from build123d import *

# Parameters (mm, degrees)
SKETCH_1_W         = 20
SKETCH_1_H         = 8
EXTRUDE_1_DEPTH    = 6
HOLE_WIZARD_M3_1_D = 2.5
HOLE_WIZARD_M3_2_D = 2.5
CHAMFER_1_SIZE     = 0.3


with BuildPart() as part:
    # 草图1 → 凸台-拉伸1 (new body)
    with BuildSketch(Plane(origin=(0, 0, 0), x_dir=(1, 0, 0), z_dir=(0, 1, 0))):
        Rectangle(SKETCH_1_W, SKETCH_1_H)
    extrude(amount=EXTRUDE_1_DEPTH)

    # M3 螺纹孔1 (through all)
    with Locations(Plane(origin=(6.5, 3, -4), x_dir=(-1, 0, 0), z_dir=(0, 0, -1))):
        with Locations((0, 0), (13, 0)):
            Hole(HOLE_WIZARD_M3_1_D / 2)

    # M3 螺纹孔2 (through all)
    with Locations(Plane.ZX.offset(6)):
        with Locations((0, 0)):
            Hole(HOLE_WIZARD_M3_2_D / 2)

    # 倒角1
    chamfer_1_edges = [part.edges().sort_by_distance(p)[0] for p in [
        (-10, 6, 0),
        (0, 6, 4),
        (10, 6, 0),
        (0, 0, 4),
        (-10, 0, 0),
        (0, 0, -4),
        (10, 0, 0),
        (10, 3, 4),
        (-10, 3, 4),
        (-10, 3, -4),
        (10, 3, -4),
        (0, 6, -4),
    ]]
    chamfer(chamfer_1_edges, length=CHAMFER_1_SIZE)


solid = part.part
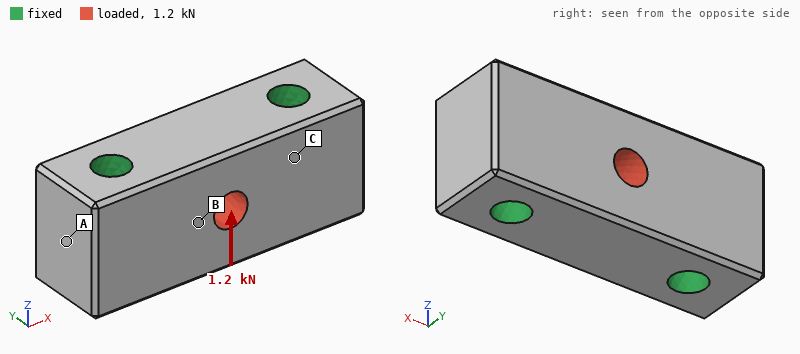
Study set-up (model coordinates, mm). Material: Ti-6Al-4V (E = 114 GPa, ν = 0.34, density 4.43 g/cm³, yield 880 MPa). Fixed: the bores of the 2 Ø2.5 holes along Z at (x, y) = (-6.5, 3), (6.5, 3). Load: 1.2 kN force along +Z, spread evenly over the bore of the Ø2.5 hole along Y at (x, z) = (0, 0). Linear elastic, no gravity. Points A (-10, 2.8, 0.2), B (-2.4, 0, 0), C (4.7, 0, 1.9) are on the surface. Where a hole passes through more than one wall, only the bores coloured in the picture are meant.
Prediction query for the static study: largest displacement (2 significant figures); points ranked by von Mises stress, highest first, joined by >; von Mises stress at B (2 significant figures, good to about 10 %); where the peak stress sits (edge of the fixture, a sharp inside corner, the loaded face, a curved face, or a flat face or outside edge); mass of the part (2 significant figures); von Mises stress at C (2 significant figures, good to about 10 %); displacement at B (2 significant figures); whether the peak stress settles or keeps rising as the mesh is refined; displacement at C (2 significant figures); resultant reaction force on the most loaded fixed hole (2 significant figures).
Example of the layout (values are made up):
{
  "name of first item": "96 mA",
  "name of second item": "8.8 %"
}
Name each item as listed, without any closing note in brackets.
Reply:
{
  "largest displacement": "2.3 µm",
  "points ranked by von Mises stress, highest first, joined by >": "B > C > A",
  "von Mises stress at B": "30 MPa",
  "where the peak stress sits": "edge of the fixture",
  "mass of the part": "3.7 g",
  "von Mises stress at C": "17 MPa",
  "displacement at B": "1.4 µm",
  "whether the peak stress settles or keeps rising as the mesh is refined": "keeps rising",
  "displacement at C": "0.51 µm",
  "resultant reaction force on the most loaded fixed hole": "600 N"
}
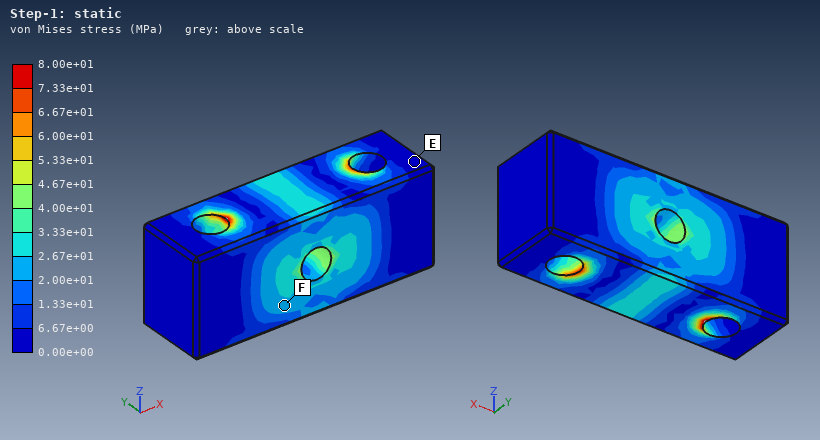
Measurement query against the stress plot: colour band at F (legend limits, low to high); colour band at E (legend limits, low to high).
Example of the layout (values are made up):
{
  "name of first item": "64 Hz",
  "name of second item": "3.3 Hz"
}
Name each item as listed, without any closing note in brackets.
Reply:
{
  "colour band at F": "2.00e+01 to 2.67e+01 MPa",
  "colour band at E": "0.00e+00 to 6.67e+00 MPa"
}
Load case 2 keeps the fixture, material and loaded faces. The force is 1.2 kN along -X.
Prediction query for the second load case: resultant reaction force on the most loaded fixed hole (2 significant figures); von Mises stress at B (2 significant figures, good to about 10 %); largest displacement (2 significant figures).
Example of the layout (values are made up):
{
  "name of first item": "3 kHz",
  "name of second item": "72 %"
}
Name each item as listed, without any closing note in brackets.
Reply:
{
  "resultant reaction force on the most loaded fixed hole": "600 N",
  "von Mises stress at B": "23 MPa",
  "largest displacement": "0.89 µm"
}
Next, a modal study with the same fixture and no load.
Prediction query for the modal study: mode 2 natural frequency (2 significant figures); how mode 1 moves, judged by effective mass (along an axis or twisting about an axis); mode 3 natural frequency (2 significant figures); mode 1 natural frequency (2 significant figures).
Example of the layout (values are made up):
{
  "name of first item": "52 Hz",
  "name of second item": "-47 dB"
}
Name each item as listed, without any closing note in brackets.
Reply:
{
  "mode 2 natural frequency": "120 kHz",
  "how mode 1 moves, judged by effective mass": "along Y",
  "mode 3 natural frequency": "120 kHz",
  "mode 1 natural frequency": "98 kHz"
}
